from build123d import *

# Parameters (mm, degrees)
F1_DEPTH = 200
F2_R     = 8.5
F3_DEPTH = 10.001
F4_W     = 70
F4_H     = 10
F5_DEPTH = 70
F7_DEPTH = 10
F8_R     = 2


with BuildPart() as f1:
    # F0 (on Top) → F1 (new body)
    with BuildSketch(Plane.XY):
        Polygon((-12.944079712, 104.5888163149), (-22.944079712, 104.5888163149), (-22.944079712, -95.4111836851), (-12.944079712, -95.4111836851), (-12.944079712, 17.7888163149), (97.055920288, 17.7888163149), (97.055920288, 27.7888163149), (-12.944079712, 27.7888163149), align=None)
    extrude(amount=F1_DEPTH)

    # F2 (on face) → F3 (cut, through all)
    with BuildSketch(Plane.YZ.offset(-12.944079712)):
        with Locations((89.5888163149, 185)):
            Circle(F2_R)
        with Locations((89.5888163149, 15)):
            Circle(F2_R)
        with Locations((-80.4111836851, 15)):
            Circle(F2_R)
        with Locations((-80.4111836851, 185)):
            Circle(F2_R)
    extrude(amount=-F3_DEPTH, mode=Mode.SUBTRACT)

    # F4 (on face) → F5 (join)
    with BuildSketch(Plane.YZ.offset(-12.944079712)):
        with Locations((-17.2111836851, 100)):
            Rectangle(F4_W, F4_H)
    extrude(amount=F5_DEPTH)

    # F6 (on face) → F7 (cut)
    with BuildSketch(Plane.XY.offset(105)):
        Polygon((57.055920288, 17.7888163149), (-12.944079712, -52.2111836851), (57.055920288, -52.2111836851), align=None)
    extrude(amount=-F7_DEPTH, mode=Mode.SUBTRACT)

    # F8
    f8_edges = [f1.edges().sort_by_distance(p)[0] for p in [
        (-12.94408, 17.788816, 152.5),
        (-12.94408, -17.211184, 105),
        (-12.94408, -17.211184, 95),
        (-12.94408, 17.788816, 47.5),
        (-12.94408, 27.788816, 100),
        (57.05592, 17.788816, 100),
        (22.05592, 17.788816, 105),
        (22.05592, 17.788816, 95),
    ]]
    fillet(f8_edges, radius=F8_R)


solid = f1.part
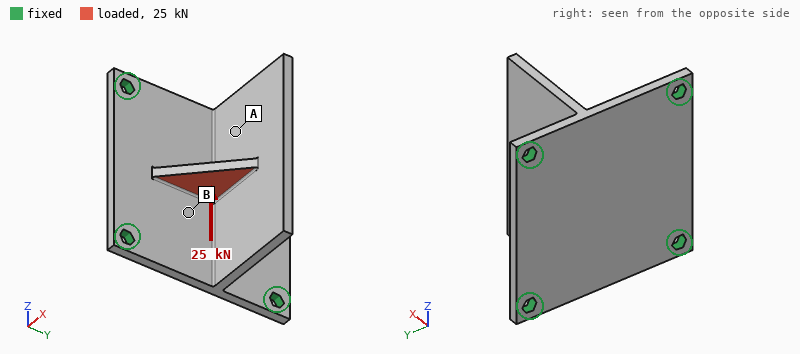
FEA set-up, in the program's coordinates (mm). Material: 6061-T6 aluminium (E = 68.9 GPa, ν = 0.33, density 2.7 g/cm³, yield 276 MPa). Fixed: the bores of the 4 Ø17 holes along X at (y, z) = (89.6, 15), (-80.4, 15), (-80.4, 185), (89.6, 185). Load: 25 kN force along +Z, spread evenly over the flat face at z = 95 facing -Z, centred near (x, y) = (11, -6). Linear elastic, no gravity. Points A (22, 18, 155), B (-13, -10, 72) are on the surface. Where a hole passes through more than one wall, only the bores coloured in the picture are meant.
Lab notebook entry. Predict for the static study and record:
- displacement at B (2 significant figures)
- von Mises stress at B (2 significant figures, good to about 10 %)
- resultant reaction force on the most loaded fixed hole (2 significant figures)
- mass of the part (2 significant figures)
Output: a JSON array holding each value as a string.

["0.088 mm", "31 MPa", "7.8 kN", "1.7 kg"]
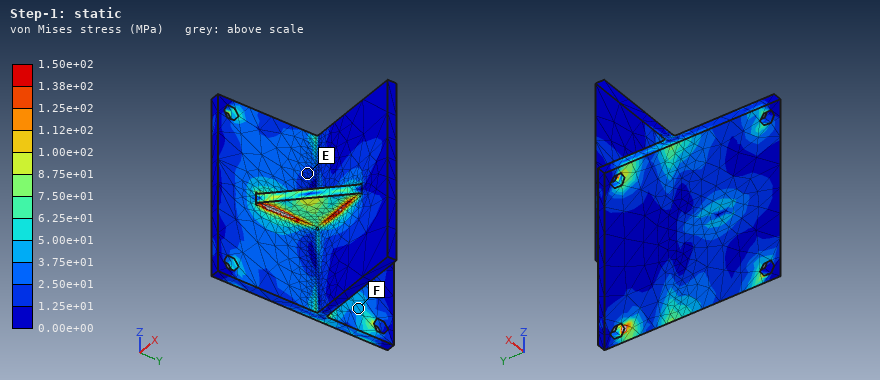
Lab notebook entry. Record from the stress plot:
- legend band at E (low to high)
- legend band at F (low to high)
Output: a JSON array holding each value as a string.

["1.25e+01 to 2.50e+01 MPa", "3.75e+01 to 5.00e+01 MPa"]
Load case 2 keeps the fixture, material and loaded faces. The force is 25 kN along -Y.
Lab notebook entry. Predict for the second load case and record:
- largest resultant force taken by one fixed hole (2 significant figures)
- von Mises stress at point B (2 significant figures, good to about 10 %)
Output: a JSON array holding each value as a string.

["7.7 kN", "43 MPa"]
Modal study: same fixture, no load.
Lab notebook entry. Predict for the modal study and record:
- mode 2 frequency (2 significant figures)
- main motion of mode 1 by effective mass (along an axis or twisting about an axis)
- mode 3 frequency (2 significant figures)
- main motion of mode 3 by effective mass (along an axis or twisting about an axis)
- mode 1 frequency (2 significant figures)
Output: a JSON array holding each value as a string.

["970 Hz", "along Y", "1000 Hz", "along X", "870 Hz"]
